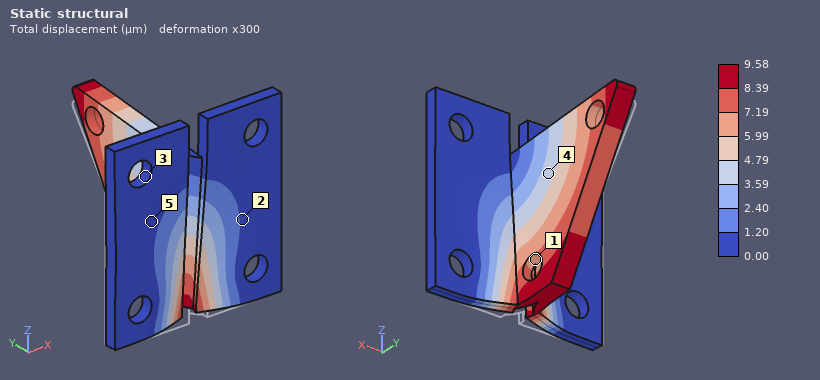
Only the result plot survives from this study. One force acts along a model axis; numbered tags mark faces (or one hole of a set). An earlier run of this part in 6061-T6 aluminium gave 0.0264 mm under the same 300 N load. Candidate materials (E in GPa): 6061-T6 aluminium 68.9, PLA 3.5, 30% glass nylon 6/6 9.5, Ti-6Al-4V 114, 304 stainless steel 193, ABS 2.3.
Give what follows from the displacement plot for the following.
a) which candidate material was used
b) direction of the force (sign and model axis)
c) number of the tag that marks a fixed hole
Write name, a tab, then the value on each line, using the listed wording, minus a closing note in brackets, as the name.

which candidate material was used	304 stainless steel
direction of the force	+Y
number of the tag that marks a fixed hole	3
